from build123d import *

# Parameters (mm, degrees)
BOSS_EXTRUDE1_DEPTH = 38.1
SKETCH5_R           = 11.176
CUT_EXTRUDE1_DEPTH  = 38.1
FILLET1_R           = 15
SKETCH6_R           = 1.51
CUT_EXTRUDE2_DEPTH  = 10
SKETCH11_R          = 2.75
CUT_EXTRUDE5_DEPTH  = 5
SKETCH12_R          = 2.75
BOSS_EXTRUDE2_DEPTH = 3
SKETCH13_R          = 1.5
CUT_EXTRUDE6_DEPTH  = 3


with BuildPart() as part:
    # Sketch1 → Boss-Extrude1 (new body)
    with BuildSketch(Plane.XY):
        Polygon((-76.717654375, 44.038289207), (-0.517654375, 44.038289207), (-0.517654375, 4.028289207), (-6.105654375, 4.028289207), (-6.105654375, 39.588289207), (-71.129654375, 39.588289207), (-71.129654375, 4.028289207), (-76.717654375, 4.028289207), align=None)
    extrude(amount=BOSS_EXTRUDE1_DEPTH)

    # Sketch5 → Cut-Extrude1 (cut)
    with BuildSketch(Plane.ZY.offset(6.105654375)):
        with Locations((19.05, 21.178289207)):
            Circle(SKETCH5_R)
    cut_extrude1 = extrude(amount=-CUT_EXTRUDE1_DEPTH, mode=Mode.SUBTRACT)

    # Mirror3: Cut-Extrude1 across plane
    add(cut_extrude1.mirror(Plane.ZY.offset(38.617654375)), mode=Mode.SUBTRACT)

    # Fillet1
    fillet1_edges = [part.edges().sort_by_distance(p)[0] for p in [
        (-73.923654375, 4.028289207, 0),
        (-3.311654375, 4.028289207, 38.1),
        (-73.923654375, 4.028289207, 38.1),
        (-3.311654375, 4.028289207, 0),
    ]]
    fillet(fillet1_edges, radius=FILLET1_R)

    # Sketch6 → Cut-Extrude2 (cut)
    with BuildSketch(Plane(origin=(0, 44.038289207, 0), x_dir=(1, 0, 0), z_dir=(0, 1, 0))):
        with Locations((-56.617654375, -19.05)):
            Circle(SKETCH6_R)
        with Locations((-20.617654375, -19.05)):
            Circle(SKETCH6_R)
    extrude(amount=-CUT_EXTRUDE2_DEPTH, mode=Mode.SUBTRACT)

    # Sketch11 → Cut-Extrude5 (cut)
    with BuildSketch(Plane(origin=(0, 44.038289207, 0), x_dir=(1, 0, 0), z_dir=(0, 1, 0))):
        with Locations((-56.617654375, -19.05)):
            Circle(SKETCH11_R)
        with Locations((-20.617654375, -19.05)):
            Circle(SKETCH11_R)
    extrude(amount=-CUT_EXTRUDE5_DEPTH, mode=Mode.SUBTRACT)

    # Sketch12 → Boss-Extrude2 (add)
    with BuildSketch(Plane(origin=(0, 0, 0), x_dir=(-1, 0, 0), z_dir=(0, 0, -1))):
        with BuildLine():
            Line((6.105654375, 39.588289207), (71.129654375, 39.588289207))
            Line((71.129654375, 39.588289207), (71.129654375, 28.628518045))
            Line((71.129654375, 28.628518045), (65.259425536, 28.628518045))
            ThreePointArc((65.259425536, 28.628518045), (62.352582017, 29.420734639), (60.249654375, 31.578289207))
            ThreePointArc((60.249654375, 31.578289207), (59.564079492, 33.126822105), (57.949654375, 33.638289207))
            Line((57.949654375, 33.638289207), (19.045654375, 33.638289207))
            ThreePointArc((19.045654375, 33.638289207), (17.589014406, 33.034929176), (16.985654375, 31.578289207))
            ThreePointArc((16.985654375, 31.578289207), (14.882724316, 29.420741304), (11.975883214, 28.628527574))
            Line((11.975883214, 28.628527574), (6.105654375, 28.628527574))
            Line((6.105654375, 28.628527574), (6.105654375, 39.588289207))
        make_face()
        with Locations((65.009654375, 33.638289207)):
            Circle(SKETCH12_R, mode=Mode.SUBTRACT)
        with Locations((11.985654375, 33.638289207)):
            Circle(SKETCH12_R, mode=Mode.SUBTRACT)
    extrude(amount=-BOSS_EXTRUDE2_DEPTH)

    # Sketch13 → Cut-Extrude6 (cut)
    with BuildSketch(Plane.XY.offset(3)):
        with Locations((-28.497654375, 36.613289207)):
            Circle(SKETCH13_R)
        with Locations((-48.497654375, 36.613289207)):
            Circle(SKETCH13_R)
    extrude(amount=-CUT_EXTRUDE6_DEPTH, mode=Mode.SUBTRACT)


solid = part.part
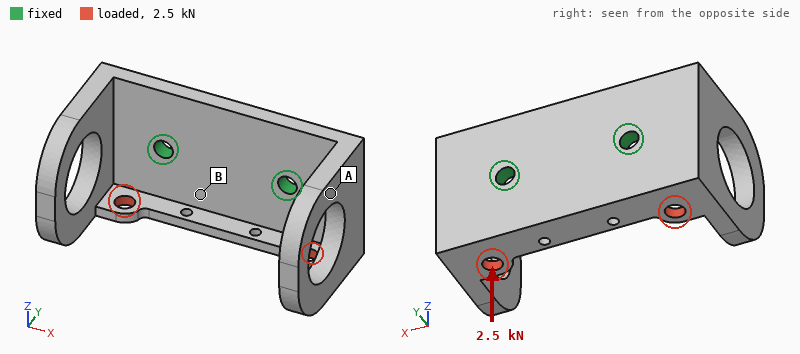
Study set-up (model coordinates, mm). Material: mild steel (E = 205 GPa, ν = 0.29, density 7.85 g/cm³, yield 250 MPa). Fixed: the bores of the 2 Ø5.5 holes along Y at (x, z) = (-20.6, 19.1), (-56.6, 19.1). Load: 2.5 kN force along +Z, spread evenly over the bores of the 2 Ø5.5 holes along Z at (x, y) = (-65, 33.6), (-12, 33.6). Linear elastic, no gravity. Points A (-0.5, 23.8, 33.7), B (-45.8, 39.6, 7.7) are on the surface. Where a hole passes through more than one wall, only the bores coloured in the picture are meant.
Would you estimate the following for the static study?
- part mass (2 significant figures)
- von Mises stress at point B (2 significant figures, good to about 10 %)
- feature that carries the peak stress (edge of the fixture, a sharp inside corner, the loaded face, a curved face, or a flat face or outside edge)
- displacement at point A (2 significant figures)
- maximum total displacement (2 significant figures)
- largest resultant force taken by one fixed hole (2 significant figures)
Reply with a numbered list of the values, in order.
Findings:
1. 190 g
2. 29 MPa
3. the loaded face
4. 36 µm
5. 59 µm
6. 1.3 kN
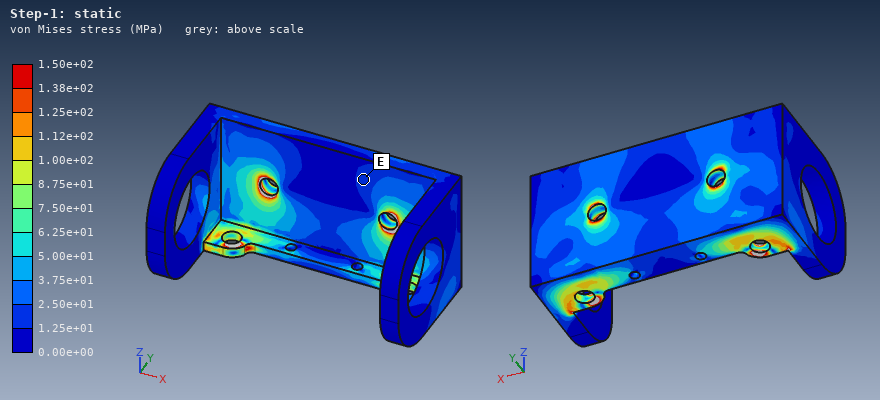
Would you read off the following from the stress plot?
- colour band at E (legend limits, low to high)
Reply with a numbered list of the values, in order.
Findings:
1. 1.25e+01 to 2.50e+01 MPa
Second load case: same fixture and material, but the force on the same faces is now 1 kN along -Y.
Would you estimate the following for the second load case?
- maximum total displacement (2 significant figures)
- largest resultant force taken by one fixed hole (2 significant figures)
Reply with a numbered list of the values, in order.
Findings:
1. 40 µm
2. 520 N
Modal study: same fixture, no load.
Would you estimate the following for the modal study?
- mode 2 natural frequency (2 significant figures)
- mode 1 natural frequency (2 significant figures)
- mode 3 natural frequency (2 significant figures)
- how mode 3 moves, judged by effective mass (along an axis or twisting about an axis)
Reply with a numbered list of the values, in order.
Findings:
1. 2200 Hz
2. 2200 Hz
3. 2600 Hz
4. along Z
